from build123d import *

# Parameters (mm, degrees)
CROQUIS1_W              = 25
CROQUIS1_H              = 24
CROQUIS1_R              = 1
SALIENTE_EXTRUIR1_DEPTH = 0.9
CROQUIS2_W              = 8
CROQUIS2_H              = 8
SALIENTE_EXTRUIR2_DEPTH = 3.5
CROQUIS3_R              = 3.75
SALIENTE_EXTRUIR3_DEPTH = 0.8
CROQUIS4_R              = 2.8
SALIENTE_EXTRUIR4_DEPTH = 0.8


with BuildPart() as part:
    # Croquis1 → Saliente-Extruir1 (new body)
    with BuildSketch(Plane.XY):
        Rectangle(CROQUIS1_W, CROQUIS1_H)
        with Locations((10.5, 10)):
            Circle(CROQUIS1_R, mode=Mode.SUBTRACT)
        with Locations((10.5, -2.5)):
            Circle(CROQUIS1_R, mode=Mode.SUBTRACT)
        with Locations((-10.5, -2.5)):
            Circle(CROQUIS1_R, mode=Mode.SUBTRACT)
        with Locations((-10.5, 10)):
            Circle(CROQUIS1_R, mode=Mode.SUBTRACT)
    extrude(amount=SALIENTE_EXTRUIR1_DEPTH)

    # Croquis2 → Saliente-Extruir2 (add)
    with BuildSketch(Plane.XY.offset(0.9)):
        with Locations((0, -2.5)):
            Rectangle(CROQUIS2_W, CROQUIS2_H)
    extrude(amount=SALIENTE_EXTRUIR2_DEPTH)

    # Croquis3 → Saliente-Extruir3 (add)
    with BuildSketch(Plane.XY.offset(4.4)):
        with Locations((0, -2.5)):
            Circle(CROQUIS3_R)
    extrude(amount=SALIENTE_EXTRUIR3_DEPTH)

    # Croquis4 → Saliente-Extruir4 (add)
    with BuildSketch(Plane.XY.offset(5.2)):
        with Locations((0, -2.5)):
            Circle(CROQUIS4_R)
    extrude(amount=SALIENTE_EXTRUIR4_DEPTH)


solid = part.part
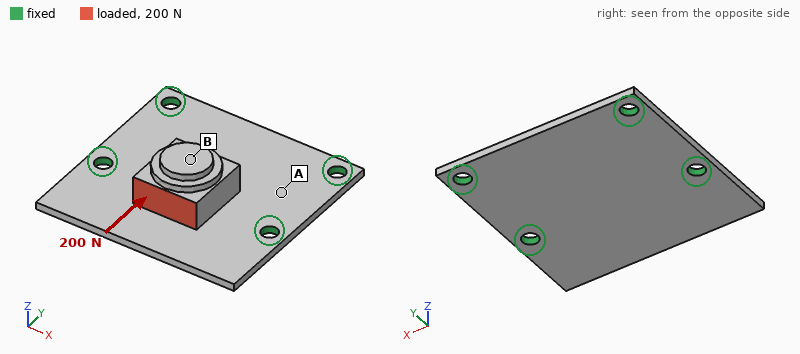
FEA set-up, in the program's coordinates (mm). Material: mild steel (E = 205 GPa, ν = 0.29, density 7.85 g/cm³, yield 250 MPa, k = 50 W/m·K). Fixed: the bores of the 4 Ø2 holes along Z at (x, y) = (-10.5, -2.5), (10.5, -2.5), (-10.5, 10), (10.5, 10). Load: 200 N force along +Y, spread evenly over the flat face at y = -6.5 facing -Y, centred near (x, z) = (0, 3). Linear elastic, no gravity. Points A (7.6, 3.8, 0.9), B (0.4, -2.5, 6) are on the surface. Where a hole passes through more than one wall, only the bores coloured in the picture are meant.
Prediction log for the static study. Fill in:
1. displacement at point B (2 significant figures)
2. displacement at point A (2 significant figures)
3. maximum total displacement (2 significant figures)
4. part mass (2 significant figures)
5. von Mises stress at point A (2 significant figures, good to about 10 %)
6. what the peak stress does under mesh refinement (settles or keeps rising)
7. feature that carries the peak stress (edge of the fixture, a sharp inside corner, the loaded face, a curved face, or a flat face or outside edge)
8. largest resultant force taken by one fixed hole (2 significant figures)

13 µm
3.6 µm
23 µm
6.3 g
29 MPa
keeps rising
edge of the fixture
64 N
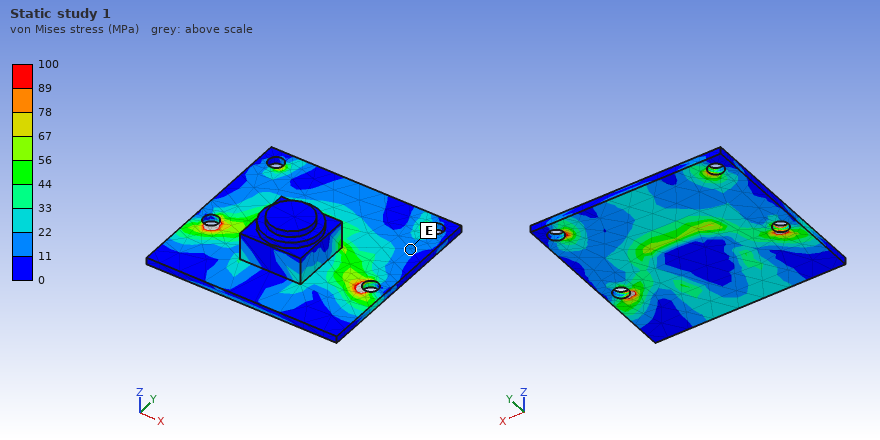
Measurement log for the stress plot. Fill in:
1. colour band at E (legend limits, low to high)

11 to 22 MPa
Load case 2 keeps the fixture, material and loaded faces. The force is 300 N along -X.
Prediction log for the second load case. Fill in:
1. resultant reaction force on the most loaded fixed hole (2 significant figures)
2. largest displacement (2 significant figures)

140 N
7.0 µm
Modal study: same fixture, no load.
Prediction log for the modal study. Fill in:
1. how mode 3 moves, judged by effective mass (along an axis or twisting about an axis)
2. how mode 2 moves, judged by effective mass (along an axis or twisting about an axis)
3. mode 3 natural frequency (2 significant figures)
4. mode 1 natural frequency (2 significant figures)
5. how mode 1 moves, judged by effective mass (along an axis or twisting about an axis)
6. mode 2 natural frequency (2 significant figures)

twisting about Y
along Z
13 kHz
6800 Hz
along Z
9700 Hz
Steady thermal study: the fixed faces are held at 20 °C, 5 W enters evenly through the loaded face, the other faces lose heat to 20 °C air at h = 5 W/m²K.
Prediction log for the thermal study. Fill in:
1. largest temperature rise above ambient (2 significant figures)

40 K
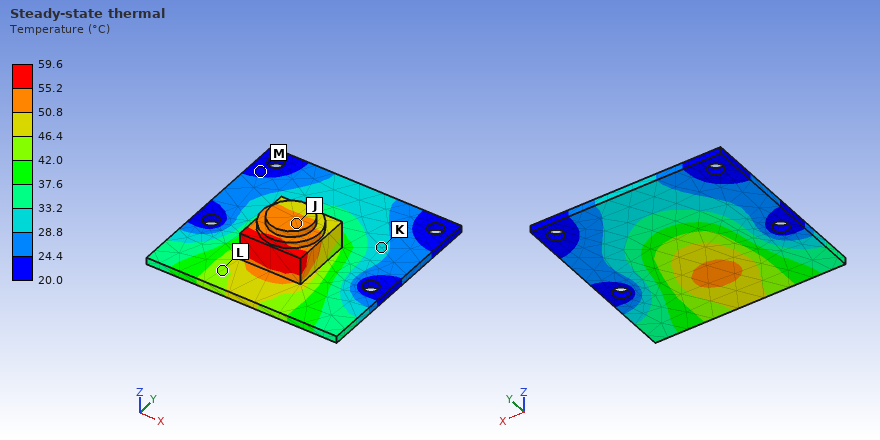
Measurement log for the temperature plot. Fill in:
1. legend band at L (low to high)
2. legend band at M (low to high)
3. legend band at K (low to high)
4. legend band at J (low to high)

42.0 to 46.4 °C
20.0 to 24.4 °C
28.8 to 33.2 °C
50.8 to 55.2 °C
